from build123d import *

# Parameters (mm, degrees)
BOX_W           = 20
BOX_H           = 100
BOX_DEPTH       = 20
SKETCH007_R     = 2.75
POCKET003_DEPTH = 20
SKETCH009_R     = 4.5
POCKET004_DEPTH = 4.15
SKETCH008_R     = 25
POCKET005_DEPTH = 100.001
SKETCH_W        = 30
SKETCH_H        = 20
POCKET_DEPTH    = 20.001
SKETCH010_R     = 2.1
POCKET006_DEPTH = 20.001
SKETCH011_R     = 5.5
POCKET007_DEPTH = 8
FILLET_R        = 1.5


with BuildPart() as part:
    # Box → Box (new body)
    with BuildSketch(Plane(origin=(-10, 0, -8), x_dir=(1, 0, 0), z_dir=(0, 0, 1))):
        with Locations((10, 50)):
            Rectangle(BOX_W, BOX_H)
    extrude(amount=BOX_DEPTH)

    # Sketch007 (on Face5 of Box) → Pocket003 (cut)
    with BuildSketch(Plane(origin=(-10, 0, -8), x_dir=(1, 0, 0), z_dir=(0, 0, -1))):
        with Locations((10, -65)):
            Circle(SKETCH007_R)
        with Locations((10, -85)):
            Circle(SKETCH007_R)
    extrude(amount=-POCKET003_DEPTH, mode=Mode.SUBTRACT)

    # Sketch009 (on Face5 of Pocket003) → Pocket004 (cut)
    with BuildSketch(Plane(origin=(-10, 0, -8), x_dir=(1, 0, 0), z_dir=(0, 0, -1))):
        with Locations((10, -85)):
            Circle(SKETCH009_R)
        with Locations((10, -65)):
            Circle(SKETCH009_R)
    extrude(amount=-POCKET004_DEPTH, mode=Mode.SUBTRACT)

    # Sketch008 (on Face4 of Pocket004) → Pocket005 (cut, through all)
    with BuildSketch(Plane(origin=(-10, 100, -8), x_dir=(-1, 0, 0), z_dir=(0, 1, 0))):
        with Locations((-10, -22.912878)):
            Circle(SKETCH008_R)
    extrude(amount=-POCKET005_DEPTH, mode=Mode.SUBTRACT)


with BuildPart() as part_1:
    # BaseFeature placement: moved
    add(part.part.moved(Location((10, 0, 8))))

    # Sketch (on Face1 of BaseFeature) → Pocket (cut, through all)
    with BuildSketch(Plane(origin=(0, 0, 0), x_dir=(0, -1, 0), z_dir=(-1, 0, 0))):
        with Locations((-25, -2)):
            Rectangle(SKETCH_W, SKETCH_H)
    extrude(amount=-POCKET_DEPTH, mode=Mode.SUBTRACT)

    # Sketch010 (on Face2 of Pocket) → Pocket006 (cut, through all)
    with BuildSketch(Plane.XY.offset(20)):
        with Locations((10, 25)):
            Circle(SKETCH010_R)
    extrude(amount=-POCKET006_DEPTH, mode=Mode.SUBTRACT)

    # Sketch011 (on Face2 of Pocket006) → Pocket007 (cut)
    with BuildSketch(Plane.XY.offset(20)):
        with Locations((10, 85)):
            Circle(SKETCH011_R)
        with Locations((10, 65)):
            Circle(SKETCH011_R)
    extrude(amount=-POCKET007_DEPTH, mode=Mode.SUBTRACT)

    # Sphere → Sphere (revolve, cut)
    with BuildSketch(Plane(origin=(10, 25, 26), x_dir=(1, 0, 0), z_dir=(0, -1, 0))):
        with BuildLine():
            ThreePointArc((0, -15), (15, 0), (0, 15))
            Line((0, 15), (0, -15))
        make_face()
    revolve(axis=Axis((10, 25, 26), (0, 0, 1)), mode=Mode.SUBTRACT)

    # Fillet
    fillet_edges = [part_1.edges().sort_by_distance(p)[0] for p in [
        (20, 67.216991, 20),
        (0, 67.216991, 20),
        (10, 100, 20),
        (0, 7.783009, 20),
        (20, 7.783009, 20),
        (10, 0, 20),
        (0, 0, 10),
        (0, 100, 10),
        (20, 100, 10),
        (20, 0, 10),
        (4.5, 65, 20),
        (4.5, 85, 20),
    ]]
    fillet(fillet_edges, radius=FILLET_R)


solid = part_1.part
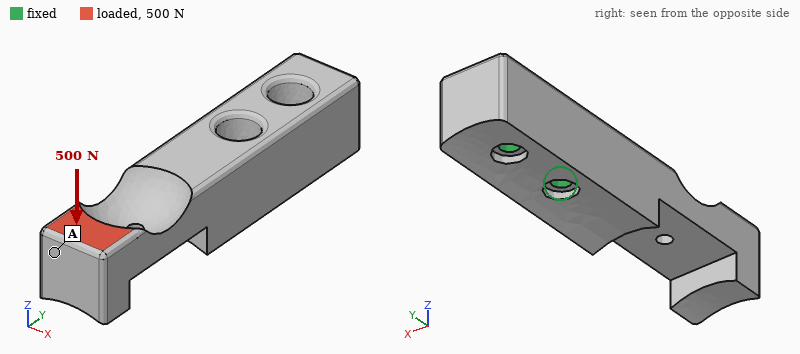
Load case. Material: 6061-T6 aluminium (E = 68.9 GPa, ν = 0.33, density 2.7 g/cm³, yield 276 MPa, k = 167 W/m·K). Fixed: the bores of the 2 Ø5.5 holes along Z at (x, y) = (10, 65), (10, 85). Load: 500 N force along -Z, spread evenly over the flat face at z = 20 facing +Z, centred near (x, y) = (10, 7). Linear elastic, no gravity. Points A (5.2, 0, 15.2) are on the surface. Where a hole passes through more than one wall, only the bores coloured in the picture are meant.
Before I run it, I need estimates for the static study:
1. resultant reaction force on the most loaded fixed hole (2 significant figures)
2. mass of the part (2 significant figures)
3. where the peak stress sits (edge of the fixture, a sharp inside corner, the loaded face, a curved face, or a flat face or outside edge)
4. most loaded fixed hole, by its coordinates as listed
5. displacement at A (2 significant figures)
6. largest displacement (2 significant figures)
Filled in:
1.5 kN
76 g
a curved face
(10, 65)
0.39 mm
0.41 mm
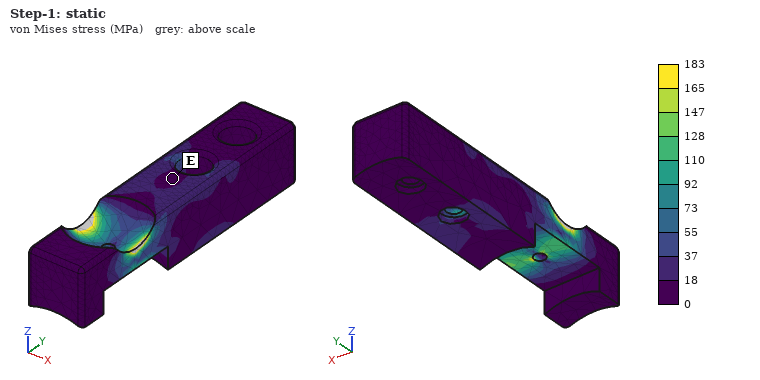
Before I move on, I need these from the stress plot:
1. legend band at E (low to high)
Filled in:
0 to 18 MPa
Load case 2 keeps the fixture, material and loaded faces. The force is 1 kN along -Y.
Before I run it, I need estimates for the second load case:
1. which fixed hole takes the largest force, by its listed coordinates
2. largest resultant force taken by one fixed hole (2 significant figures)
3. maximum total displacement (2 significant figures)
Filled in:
(10, 65)
740 N
0.34 mm
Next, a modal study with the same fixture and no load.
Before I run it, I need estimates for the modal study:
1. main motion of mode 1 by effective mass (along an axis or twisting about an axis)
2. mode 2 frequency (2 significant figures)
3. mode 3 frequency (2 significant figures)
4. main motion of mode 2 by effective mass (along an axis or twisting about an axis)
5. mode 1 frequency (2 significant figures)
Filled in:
along Z
3000 Hz
5900 Hz
along X
1700 Hz
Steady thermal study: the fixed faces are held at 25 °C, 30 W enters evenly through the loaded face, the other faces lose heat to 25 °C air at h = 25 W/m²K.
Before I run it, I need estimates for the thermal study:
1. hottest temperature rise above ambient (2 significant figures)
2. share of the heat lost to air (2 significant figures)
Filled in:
63 K
13 %
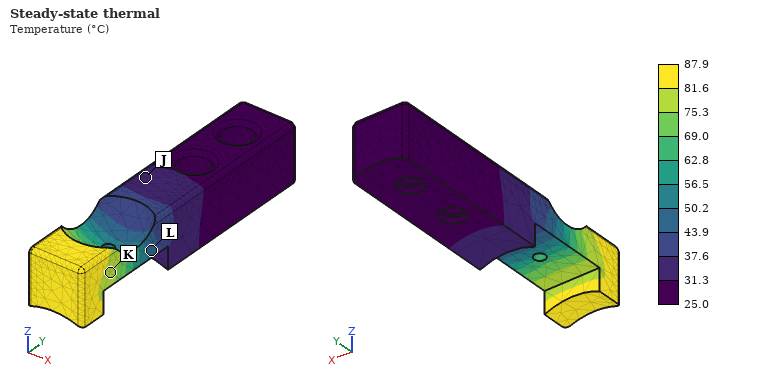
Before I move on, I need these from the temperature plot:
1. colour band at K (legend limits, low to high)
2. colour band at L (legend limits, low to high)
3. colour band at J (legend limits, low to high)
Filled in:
75.3 to 81.6 °C
43.9 to 50.2 °C
31.3 to 37.6 °C
